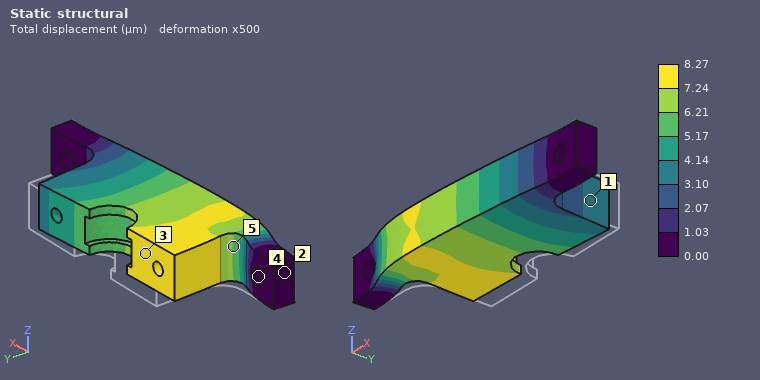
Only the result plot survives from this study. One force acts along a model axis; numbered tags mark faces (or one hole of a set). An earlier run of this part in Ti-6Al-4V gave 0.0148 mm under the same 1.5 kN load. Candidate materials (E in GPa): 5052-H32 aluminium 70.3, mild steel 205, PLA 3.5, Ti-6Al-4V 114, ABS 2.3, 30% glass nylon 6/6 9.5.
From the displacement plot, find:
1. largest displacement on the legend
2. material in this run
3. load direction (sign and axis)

8.27 µm
mild steel
-Y
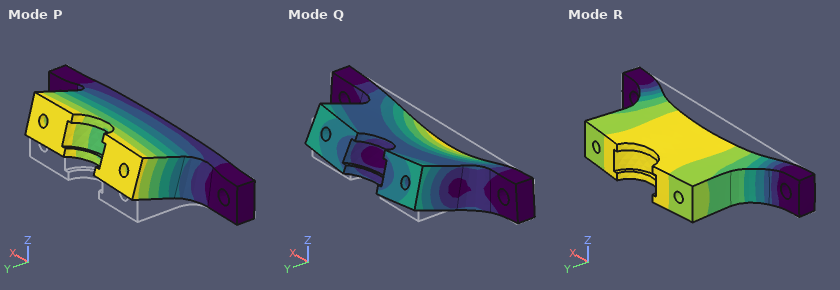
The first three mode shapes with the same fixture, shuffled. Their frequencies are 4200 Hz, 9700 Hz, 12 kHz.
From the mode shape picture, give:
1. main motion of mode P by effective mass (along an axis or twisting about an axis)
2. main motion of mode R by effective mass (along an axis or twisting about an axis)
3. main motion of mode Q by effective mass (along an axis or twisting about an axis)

along Z
along Y
along Z
